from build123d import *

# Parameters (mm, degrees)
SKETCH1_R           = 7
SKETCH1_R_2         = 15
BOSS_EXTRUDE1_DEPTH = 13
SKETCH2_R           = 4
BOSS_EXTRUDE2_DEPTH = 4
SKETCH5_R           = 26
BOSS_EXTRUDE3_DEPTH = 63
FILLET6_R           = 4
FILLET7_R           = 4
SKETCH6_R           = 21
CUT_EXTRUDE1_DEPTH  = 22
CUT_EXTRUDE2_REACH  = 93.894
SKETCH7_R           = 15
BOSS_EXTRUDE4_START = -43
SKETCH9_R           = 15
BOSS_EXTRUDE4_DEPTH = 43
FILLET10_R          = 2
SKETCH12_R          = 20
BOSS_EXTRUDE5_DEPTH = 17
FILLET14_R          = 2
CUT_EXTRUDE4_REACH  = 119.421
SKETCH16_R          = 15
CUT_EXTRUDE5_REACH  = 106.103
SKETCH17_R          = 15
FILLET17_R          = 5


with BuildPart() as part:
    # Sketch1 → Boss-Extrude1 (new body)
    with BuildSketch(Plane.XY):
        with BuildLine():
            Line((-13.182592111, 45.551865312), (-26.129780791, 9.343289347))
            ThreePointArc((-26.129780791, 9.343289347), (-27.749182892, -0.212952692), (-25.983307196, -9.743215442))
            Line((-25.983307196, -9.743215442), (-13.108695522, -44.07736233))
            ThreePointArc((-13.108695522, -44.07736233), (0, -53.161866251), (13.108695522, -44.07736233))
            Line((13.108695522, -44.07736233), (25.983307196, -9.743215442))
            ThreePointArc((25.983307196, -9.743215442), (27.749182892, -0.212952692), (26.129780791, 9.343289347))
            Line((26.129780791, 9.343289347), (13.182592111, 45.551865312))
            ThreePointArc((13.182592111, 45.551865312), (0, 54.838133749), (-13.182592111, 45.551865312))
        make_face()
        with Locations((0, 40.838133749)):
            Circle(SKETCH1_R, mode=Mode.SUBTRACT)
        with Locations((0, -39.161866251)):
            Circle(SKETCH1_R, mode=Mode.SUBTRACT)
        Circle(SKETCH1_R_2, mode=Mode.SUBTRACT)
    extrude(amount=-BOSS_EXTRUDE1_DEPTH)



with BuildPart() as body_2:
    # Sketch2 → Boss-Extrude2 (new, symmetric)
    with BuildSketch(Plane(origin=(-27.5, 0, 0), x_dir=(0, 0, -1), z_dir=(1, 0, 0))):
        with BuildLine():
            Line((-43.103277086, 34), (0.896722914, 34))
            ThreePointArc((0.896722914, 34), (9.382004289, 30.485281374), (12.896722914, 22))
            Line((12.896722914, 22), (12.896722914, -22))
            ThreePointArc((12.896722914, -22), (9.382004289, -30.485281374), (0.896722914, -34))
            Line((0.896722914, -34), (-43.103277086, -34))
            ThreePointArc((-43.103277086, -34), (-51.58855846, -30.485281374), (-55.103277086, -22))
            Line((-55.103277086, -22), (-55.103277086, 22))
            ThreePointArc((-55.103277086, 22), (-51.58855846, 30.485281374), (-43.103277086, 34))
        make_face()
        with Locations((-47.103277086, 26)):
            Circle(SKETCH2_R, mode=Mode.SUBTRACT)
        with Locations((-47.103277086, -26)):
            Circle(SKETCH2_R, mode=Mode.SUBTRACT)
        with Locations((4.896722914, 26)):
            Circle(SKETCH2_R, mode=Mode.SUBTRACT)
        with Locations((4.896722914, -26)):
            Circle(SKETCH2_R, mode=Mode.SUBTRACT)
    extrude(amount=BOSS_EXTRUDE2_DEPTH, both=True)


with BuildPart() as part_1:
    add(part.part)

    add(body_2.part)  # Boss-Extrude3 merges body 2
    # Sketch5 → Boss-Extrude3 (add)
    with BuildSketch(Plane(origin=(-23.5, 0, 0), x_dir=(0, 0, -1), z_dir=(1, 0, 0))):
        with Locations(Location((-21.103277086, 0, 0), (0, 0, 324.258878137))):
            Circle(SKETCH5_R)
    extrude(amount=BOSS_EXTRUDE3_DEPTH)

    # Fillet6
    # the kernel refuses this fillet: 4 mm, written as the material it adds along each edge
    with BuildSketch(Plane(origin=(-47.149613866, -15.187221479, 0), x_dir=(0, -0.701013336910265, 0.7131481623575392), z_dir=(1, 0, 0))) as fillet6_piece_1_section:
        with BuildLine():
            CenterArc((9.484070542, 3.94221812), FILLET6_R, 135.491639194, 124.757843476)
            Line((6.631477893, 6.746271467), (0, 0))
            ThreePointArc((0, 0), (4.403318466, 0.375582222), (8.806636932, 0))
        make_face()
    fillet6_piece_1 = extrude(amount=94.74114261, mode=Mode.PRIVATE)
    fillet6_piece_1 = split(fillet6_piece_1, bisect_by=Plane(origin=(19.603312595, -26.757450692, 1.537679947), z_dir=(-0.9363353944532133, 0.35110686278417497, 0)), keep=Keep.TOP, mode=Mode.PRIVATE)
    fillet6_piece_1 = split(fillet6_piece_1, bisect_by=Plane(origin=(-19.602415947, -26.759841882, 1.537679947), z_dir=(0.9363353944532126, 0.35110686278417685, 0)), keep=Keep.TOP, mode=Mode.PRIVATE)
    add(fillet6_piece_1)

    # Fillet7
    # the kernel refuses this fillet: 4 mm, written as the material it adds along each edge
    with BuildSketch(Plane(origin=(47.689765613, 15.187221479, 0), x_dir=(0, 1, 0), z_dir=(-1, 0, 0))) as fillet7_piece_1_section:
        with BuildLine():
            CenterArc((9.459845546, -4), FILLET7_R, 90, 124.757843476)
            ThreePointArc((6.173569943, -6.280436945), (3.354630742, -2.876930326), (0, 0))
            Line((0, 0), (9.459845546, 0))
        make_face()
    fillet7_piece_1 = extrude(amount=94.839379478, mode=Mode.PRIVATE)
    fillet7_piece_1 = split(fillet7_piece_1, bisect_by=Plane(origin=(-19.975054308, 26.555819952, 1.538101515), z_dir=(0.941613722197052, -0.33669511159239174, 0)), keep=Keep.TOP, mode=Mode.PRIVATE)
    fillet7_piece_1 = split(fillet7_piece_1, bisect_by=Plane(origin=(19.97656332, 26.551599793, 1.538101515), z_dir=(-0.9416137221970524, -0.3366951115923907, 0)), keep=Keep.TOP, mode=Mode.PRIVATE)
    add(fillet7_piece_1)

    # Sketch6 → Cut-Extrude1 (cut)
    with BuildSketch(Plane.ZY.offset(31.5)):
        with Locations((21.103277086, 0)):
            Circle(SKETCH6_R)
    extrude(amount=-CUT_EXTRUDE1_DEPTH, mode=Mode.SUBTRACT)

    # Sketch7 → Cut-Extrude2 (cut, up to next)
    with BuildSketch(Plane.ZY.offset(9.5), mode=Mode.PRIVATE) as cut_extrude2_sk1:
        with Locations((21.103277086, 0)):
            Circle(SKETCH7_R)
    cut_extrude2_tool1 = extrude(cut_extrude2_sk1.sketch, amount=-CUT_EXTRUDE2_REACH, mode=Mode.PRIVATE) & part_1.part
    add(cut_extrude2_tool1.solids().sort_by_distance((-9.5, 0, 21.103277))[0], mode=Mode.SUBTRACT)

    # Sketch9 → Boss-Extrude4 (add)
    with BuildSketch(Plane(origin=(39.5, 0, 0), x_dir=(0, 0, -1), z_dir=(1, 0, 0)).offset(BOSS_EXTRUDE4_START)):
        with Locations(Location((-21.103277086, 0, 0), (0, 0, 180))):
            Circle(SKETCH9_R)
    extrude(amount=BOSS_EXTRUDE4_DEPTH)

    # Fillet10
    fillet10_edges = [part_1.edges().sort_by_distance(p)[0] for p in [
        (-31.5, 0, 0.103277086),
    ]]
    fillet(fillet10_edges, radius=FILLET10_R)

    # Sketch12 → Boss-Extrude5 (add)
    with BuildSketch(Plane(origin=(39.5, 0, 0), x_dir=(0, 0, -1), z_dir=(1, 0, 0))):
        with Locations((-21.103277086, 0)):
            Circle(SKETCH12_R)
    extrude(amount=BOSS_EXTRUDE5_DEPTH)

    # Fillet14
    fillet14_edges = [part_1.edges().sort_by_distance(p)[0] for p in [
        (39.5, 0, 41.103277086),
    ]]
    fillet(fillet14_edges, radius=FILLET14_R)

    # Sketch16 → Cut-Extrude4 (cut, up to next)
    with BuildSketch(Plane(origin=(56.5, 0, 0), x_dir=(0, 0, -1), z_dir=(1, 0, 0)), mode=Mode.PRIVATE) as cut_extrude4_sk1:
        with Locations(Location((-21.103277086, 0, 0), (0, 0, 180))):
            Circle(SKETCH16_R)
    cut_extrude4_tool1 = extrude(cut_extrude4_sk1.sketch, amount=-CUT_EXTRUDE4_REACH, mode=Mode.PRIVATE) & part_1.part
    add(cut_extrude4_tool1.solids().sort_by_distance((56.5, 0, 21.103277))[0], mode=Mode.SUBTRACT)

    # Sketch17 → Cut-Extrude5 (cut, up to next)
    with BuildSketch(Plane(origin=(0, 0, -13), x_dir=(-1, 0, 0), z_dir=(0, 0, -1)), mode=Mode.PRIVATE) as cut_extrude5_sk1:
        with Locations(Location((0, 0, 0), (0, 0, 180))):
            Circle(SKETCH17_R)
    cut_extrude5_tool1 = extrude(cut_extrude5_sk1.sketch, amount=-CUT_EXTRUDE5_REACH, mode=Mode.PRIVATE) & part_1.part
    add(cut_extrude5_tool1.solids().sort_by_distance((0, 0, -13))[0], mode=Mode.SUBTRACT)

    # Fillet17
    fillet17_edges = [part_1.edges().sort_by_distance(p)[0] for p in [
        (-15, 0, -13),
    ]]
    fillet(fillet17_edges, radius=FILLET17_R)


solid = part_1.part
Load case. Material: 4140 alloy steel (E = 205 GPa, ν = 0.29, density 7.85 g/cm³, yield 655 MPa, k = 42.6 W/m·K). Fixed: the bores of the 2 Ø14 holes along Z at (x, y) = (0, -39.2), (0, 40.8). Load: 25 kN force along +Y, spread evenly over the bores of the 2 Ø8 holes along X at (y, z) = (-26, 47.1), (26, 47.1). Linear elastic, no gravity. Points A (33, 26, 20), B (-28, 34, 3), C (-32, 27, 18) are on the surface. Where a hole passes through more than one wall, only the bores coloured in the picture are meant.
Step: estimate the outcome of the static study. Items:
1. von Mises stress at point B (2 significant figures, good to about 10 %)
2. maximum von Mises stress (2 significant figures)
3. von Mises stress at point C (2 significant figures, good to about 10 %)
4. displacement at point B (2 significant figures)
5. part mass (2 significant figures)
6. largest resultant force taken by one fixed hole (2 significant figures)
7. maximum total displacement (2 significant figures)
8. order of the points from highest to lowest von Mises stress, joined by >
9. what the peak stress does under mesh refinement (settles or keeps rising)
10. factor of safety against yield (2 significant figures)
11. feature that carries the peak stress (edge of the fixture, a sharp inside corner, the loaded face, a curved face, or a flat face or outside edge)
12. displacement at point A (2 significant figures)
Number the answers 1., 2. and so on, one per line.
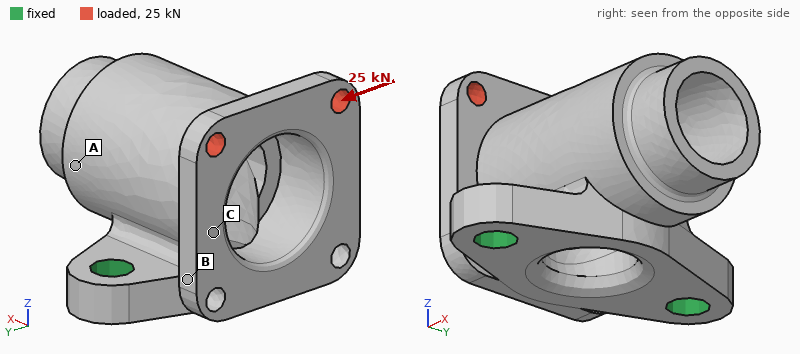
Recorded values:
1. 180 MPa
2. 530 MPa
3. 110 MPa
4. 0.087 mm
5. 1.1 kg
6. 28 kN
7. 0.27 mm
8. B > C > A
9. settles
10. 1.2
11. a curved face
12. 0.076 mm
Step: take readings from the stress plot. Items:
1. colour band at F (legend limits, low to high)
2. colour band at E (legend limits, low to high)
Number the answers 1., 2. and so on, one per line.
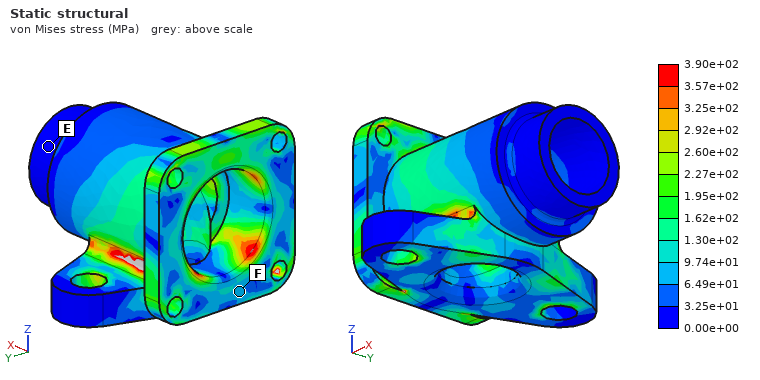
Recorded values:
1. 6.49e+01 to 9.74e+01 MPa
2. 0.00e+00 to 3.25e+01 MPa
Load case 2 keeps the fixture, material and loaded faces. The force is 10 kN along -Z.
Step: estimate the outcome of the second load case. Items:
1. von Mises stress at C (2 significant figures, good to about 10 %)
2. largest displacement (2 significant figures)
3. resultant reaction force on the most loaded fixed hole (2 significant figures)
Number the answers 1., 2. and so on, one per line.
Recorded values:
1. 34 MPa
2. 100 µm
3. 5.2 kN
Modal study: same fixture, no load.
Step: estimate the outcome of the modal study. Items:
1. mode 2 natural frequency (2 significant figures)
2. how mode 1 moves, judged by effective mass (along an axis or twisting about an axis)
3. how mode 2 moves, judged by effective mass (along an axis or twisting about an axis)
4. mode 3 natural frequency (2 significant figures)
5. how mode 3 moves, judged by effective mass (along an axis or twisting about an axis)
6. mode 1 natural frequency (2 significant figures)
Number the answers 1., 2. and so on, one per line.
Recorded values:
1. 3500 Hz
2. along X
3. along Y
4. 5700 Hz
5. along Z
6. 1900 Hz
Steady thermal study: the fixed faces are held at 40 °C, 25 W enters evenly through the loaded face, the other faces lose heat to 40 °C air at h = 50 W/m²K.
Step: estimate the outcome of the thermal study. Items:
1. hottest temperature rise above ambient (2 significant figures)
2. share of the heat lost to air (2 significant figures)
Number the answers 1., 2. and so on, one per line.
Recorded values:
1. 51 K
2. 67 %
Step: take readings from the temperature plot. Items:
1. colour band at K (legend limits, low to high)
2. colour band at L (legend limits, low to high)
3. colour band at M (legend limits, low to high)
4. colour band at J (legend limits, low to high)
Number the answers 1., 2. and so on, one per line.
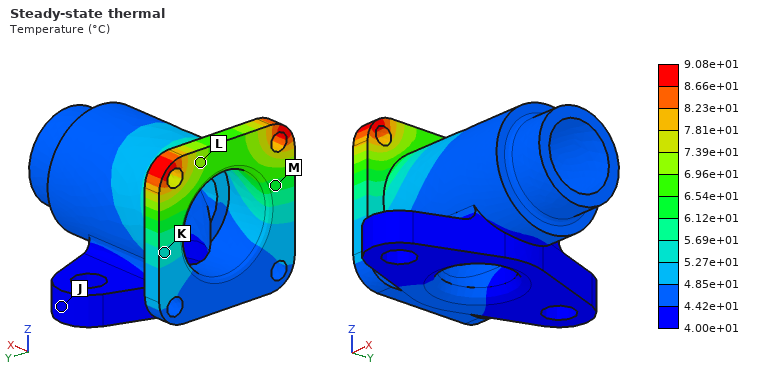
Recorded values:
1. 5.27e+01 to 5.69e+01 °C
2. 6.96e+01 to 7.39e+01 °C
3. 6.12e+01 to 6.54e+01 °C
4. 4.00e+01 to 4.42e+01 °C
